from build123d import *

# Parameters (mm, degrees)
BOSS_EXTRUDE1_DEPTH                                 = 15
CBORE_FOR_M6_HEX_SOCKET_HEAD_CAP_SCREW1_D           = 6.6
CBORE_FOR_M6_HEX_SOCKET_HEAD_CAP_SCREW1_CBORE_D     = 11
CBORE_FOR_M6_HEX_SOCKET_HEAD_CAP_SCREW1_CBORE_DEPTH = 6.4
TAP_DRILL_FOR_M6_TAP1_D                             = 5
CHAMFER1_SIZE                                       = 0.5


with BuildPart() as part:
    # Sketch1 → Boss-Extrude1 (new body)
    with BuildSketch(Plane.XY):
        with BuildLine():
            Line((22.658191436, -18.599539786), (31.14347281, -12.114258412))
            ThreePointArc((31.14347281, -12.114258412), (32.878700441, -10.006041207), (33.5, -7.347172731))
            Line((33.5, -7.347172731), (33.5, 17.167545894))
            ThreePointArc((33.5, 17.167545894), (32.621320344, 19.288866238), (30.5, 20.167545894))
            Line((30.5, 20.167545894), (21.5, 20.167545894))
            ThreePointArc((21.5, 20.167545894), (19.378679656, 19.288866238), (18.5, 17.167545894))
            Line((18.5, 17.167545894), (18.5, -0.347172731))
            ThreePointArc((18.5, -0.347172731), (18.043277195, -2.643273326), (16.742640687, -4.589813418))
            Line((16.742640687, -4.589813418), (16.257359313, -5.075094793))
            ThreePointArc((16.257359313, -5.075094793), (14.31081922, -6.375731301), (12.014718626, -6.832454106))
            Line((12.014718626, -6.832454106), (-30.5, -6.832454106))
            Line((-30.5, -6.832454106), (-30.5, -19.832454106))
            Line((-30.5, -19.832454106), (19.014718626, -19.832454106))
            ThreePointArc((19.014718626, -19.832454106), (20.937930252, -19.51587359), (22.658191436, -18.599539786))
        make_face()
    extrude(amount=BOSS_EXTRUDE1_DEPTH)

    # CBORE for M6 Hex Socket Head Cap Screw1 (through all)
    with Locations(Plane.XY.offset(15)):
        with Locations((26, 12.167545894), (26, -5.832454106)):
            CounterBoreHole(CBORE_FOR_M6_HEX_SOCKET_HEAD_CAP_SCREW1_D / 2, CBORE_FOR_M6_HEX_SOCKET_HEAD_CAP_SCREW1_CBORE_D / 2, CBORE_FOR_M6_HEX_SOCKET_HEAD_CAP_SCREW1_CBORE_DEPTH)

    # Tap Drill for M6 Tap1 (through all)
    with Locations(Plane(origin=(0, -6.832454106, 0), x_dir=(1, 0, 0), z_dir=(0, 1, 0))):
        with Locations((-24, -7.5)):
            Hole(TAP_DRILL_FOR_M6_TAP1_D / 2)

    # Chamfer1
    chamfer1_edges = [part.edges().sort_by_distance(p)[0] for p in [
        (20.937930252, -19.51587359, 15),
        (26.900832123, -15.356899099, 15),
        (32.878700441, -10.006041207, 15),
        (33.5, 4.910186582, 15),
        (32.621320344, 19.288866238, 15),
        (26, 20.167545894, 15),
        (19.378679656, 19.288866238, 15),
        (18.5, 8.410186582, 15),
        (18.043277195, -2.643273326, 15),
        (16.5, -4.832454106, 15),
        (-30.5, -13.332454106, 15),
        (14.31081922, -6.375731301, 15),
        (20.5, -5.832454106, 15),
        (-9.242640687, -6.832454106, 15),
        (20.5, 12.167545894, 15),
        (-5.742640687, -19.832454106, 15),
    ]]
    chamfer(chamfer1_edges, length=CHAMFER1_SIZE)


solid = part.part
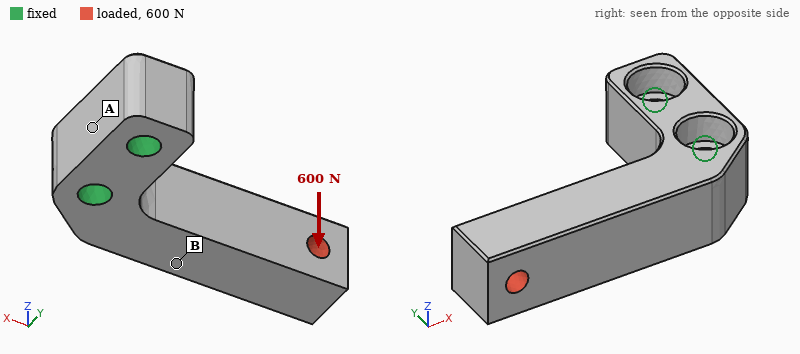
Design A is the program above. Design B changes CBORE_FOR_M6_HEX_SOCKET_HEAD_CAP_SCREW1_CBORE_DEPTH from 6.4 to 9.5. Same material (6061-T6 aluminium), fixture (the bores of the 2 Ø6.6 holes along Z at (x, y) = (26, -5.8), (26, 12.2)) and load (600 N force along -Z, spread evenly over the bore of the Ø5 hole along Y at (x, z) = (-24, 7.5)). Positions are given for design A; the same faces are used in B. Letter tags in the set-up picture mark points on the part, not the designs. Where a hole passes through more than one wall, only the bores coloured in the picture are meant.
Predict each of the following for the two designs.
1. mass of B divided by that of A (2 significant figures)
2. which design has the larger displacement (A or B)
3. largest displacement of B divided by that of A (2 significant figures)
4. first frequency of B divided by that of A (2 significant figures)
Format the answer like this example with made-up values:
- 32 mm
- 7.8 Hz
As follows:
- 0.98
- B
- 1.3
- 0.84
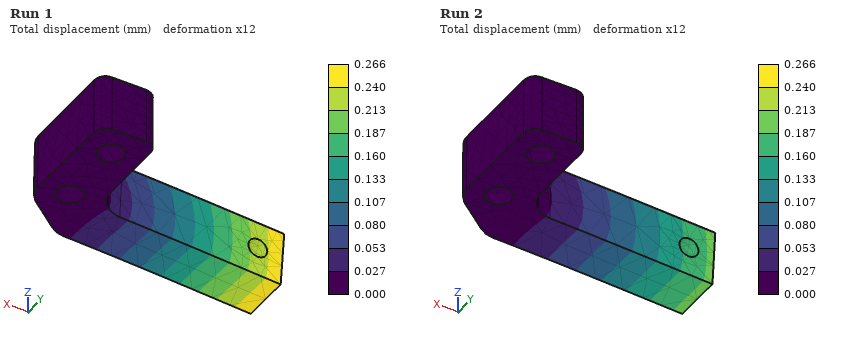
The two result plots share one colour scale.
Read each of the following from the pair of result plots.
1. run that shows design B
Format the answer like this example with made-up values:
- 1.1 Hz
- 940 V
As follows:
- Run 1
